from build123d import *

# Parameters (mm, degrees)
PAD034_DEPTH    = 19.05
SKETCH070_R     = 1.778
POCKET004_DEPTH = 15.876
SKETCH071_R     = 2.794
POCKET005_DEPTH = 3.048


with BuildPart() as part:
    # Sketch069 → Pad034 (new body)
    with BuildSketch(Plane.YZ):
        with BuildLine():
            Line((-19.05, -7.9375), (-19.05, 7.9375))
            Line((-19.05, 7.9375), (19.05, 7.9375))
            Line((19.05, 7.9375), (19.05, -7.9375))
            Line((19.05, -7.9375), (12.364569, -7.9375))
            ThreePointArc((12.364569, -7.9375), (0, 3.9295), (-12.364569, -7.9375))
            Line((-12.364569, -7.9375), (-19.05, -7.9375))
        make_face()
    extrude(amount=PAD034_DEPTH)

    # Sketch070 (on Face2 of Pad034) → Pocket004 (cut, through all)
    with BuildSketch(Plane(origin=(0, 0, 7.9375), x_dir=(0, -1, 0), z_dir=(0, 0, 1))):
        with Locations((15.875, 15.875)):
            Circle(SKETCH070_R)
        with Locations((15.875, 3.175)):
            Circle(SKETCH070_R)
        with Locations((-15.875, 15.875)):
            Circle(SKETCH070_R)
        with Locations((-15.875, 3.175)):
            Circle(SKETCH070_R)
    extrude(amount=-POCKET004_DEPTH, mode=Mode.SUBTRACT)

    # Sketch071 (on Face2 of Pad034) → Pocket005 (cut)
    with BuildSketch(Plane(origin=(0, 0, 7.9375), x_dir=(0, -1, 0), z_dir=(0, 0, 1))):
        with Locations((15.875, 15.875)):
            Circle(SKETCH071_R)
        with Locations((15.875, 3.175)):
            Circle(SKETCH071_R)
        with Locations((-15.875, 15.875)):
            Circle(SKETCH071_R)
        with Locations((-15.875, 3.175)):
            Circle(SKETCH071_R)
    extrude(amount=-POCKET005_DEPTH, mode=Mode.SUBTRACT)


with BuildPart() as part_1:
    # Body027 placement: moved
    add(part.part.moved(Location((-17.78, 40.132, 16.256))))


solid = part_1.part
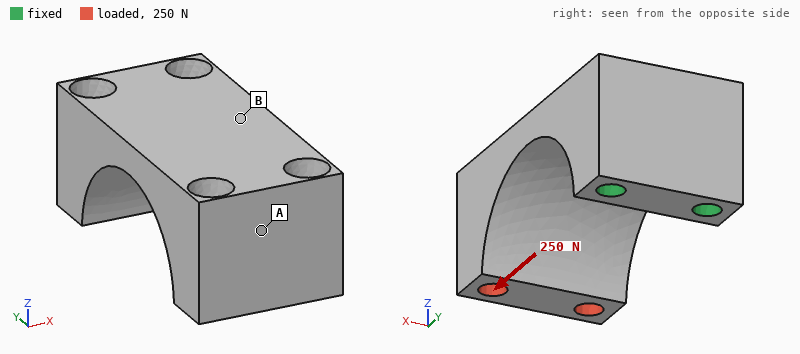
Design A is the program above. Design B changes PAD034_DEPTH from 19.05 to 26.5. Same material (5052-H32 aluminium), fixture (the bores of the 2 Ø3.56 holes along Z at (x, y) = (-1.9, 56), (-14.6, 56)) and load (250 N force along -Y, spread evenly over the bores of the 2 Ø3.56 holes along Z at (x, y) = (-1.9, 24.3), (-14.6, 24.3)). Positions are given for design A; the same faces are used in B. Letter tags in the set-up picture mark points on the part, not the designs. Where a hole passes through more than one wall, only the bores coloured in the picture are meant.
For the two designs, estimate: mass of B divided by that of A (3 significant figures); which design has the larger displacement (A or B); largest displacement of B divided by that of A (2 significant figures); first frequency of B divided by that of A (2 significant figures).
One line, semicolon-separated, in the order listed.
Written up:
1.44; A; 0.72; 0.98
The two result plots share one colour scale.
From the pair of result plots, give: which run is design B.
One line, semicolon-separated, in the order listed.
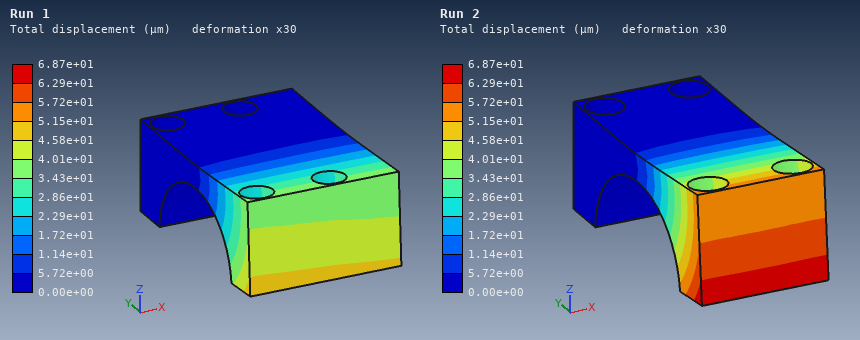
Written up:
Run 1
